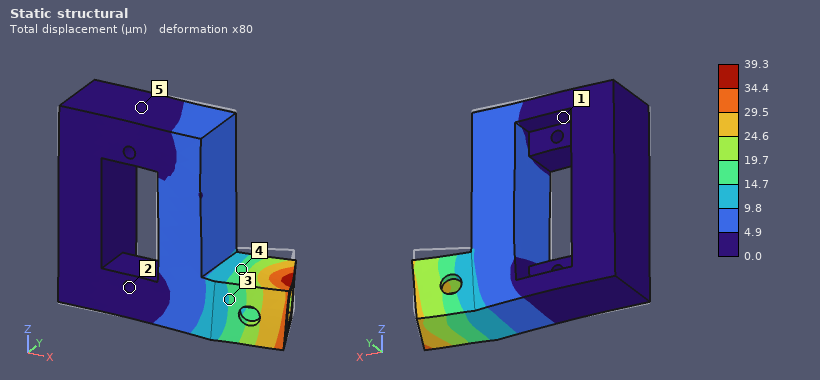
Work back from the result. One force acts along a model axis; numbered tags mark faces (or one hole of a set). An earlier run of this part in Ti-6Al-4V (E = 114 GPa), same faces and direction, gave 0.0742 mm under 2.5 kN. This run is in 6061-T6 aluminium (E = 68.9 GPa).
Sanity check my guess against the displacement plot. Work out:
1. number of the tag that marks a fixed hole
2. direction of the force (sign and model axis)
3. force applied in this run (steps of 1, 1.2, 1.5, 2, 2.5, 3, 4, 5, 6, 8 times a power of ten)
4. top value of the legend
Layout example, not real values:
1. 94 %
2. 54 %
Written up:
1. 2
2. -Z
3. 800 N
4. 39.3 µm
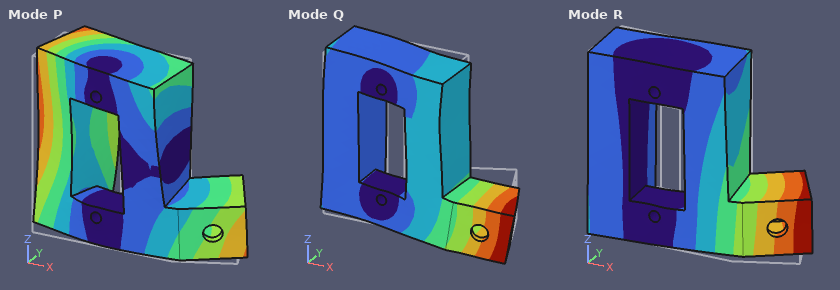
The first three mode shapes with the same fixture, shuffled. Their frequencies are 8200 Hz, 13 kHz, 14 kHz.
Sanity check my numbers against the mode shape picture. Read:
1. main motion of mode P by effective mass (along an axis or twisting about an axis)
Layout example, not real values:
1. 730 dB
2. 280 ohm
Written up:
1. along Y
